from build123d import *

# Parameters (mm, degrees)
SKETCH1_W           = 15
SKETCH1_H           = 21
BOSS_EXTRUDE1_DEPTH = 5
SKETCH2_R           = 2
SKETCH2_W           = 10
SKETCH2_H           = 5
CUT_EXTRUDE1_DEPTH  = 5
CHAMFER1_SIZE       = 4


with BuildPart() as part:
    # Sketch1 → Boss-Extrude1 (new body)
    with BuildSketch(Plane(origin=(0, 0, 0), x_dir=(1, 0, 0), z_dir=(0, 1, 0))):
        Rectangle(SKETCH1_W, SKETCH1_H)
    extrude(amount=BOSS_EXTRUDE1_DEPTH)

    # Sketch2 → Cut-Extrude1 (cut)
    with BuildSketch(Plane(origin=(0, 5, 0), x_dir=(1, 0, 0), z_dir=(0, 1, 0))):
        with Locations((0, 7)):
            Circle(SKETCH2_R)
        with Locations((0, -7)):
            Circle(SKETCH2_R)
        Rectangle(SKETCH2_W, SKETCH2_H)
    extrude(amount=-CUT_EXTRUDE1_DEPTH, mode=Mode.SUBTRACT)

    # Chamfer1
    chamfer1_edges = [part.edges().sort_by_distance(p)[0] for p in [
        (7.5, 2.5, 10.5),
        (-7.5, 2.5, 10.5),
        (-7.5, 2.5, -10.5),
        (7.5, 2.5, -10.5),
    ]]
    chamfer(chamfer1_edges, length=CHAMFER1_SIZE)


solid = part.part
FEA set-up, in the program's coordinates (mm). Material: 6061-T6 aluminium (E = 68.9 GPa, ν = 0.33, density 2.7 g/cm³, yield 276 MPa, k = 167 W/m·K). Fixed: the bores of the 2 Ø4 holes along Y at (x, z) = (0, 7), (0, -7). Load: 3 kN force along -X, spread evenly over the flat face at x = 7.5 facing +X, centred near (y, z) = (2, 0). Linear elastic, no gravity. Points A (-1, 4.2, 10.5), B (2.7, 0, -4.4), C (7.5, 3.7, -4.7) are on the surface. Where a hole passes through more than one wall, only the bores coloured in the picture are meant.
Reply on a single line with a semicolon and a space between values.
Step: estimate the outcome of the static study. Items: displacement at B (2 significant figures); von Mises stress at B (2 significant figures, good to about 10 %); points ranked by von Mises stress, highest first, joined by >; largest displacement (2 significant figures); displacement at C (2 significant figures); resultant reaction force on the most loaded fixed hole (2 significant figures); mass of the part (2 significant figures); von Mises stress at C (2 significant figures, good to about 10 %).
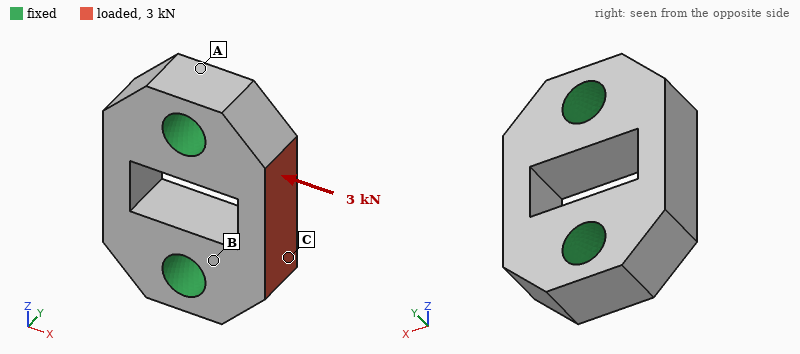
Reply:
2.6 µm; 76 MPa; B > C > A; 15 µm; 6.2 µm; 1.6 kN; 2.8 g; 46 MPa
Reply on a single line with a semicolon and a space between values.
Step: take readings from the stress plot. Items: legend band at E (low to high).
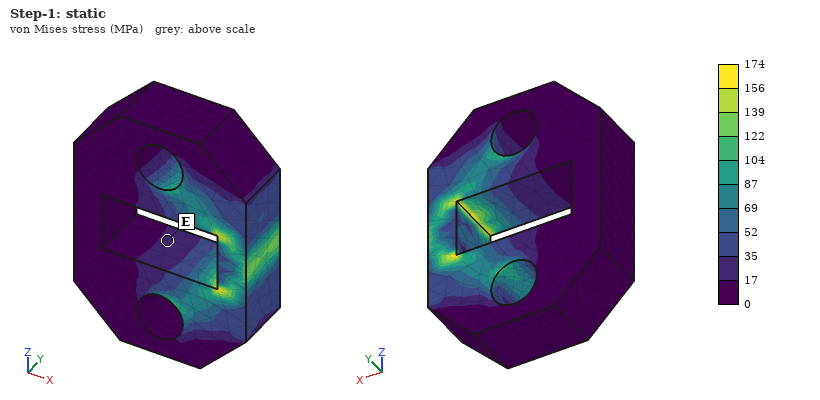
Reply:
17 to 35 MPa
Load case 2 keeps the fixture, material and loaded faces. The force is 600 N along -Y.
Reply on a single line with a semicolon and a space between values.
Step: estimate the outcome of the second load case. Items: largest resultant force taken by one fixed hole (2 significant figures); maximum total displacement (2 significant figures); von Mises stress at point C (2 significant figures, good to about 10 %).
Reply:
300 N; 13 µm; 34 MPa
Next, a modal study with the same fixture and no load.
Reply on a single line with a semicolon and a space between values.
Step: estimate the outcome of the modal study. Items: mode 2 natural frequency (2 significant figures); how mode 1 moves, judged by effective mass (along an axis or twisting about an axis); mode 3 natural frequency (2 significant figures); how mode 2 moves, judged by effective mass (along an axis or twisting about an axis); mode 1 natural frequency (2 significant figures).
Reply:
66 kHz; twisting about Z; 79 kHz; along Y; 63 kHz
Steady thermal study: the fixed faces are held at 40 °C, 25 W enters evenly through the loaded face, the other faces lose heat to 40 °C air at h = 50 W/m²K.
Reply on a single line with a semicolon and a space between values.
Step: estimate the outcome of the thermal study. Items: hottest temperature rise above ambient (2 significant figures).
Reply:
21 K
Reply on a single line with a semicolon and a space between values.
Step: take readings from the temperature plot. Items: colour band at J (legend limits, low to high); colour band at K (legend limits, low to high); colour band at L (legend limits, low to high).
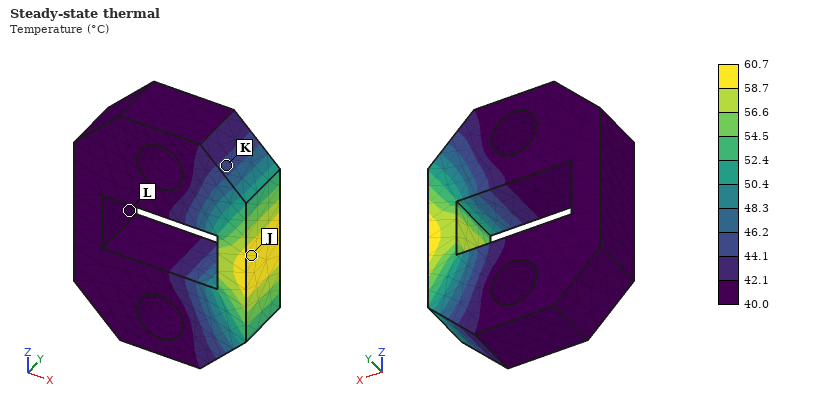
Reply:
58.7 to 60.7 °C; 44.1 to 46.2 °C; 40.0 to 42.1 °C
